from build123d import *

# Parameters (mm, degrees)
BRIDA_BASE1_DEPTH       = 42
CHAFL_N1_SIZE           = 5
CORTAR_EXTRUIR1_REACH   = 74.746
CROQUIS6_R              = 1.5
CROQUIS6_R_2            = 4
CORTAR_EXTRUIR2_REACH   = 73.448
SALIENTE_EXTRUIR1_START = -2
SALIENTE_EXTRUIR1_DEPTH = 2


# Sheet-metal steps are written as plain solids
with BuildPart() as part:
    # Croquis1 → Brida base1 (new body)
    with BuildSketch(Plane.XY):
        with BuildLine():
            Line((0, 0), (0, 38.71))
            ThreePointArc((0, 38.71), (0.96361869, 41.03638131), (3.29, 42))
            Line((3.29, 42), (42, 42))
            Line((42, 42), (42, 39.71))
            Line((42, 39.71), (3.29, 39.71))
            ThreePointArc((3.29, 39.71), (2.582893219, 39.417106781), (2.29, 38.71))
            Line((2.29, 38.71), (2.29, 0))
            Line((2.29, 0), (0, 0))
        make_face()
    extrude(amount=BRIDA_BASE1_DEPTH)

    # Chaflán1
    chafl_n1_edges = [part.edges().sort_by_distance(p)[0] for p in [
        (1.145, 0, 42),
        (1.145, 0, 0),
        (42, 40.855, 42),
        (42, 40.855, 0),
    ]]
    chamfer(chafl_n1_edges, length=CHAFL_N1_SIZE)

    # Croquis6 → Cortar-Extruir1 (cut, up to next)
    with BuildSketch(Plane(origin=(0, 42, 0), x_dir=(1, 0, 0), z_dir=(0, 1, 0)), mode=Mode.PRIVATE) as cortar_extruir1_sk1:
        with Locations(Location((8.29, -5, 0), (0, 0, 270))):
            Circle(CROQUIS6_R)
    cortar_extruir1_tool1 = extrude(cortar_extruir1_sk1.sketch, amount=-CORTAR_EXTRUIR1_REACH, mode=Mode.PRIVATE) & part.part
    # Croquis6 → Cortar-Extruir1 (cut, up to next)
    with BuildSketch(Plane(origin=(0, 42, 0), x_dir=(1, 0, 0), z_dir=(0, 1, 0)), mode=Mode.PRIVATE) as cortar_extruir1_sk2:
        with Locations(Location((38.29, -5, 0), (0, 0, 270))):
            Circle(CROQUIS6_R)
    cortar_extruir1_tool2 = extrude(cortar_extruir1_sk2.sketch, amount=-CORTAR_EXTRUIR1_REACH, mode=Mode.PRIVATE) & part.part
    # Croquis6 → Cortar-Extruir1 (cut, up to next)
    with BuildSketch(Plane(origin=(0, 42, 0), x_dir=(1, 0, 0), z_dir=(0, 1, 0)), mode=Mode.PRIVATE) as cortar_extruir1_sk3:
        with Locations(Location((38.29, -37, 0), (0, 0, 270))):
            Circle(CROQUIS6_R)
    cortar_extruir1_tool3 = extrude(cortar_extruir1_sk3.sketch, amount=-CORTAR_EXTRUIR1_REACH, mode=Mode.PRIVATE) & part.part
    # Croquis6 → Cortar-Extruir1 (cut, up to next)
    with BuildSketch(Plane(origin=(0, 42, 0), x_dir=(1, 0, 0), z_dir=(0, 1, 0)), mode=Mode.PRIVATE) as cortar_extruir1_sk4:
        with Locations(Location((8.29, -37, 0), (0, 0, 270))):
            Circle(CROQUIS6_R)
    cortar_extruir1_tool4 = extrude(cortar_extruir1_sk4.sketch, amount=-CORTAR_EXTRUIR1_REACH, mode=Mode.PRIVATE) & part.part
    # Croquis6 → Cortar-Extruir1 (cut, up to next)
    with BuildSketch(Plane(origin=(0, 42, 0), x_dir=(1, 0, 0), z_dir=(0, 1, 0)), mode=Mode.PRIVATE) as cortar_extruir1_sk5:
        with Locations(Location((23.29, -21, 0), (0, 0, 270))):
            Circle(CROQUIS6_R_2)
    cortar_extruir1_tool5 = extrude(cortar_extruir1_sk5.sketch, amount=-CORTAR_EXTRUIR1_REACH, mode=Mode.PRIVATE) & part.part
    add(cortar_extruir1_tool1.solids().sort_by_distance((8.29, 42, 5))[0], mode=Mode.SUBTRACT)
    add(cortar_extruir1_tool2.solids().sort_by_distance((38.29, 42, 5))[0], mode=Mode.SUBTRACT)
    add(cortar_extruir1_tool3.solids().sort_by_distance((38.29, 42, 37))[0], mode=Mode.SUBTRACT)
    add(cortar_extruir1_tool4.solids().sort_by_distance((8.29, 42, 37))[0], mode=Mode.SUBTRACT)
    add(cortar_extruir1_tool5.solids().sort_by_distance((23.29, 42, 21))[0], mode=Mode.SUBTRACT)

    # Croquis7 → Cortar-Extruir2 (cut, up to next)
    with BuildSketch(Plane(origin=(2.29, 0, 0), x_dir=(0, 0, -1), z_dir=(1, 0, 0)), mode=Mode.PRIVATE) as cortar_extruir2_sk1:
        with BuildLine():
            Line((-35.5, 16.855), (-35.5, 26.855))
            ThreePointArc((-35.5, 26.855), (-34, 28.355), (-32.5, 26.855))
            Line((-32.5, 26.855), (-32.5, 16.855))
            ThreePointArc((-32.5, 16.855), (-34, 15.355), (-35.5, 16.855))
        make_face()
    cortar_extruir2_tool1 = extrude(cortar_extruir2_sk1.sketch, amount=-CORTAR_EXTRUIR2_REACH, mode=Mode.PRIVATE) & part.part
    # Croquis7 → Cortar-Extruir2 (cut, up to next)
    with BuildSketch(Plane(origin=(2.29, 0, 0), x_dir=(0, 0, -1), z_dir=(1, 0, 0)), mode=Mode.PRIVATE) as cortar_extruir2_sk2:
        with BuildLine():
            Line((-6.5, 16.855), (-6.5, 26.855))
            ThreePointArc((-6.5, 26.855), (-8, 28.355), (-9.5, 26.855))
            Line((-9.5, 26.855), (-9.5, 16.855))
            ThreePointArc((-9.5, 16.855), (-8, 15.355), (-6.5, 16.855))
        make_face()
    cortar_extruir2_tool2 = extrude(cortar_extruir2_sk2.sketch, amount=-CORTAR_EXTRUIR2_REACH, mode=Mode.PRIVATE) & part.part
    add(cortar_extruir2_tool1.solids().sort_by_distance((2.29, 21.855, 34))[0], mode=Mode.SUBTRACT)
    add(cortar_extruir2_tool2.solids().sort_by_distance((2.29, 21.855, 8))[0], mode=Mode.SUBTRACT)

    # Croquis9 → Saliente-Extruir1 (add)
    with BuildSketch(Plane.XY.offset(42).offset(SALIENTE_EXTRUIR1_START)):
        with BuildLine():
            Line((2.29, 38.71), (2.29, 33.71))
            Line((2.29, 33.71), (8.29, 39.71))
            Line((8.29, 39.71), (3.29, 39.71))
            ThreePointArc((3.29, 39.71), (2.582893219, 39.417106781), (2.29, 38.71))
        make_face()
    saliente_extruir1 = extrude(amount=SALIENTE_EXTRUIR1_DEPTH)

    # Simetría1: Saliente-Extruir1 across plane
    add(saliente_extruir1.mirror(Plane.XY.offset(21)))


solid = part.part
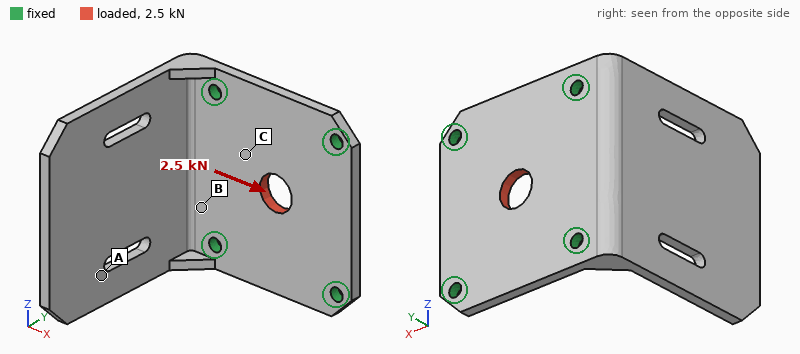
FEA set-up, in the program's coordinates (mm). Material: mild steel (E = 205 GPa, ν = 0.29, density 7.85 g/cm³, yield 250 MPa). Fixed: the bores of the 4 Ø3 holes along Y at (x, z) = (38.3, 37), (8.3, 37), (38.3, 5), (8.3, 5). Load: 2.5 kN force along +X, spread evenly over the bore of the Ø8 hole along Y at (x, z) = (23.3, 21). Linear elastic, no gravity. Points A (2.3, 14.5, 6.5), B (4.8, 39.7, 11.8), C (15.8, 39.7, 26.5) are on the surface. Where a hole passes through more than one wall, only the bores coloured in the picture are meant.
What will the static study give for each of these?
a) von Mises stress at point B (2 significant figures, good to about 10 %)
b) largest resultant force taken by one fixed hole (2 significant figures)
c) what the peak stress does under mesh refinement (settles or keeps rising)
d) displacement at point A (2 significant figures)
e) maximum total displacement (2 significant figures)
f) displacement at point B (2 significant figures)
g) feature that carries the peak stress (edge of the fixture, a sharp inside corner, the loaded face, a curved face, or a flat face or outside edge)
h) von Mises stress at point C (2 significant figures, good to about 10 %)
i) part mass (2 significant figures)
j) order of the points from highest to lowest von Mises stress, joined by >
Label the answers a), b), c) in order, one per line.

a) 16 MPa
b) 710 N
c) keeps rising
d) 1.5 µm
e) 4.0 µm
f) 1.4 µm
g) edge of the fixture
h) 31 MPa
i) 58 g
j) C > B > A
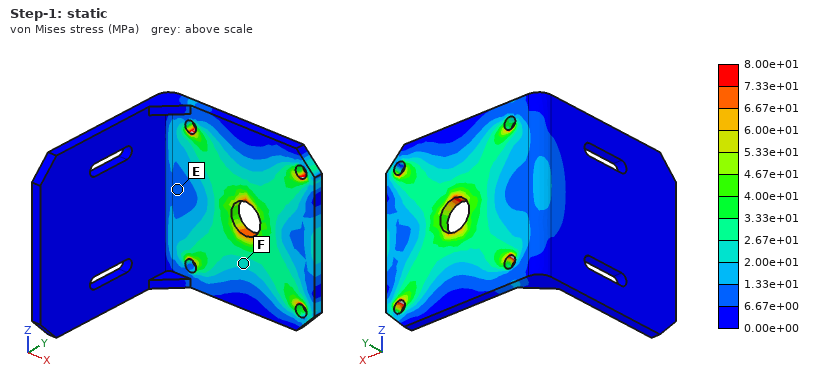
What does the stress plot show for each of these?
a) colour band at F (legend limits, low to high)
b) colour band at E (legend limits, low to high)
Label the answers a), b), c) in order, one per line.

a) 2.00e+01 to 2.67e+01 MPa
b) 6.67e+00 to 1.33e+01 MPa
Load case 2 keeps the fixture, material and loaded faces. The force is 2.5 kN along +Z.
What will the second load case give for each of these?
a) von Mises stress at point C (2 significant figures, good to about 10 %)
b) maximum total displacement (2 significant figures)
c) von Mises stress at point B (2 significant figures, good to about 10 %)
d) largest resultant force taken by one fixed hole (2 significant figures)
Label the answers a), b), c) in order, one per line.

a) 29 MPa
b) 3.7 µm
c) 8.1 MPa
d) 700 N
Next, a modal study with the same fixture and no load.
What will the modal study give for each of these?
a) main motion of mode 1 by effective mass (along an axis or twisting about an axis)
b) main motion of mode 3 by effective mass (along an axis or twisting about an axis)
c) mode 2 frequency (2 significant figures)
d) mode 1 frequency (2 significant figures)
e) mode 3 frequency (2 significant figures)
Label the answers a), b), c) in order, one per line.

a) along X
b) along Z
c) 2700 Hz
d) 1000 Hz
e) 5100 Hz
